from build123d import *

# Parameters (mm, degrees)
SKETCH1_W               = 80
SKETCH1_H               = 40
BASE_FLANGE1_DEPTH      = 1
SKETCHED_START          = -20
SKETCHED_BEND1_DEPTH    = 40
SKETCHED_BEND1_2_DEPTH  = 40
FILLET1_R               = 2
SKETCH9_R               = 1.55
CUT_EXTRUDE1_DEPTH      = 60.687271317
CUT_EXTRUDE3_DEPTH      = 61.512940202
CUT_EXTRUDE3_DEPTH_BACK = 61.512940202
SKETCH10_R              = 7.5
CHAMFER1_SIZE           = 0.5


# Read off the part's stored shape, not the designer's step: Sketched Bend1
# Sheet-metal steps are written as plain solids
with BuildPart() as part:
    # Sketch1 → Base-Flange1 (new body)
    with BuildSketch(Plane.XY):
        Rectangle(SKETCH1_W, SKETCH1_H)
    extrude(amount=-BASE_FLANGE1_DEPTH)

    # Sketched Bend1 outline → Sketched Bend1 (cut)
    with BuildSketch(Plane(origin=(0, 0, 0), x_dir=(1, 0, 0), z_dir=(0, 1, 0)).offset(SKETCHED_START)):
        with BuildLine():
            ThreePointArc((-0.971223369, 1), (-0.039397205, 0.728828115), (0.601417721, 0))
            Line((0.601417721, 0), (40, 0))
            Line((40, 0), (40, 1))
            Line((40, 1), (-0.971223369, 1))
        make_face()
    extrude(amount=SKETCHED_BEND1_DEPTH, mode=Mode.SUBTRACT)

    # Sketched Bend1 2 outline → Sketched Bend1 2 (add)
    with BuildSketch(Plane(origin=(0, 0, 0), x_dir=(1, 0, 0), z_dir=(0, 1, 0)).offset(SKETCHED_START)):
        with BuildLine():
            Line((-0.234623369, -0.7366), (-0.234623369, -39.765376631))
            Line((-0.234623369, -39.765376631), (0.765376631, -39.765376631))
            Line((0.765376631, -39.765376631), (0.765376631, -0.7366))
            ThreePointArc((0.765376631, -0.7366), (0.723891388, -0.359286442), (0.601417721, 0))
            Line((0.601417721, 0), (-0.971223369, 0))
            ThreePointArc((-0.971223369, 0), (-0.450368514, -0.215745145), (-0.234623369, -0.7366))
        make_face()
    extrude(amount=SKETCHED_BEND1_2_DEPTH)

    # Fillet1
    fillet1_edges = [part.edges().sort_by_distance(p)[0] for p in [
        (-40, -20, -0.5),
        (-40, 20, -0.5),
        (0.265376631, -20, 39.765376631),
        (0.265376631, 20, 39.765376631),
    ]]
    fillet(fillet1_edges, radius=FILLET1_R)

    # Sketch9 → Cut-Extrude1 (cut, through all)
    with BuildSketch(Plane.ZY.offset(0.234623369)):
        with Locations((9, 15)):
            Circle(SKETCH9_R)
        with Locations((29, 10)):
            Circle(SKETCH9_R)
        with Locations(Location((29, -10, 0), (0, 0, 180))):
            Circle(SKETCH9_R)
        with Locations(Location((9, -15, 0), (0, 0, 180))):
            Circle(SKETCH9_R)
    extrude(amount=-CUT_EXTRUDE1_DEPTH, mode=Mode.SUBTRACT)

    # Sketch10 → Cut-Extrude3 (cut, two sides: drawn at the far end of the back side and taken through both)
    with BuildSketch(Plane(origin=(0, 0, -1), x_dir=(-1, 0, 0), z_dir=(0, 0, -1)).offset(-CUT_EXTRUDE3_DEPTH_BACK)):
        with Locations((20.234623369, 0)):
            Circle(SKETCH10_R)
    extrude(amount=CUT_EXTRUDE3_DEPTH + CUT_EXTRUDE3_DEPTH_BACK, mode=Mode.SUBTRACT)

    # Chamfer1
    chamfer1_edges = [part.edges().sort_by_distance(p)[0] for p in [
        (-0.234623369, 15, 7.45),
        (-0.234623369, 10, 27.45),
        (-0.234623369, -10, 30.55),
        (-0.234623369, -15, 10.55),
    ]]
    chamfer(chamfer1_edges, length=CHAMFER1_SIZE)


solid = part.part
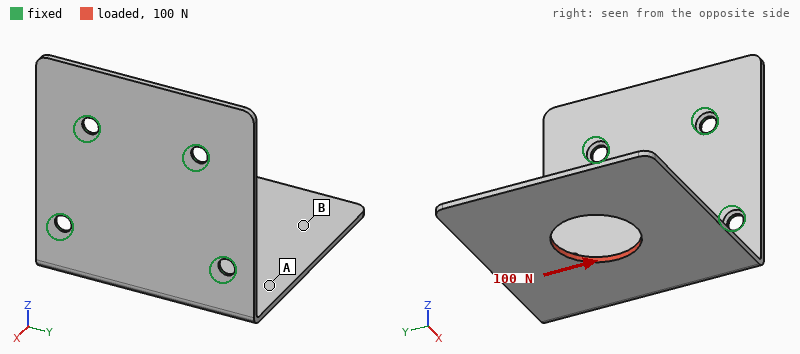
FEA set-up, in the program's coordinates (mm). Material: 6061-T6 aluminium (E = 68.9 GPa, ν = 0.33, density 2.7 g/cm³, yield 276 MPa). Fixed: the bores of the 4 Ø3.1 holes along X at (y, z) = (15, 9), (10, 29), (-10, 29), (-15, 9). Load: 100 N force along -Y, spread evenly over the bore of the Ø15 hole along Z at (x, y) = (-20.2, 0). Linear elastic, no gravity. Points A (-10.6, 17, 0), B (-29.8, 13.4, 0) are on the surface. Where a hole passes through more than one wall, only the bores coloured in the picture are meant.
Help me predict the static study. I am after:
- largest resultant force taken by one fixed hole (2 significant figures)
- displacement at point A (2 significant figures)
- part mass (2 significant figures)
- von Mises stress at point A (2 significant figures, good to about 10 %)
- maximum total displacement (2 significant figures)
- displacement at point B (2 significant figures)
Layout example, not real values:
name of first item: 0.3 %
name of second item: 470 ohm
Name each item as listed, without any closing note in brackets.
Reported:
largest resultant force taken by one fixed hole: 96 N
displacement at point A: 0.23 mm
part mass: 8.1 g
von Mises stress at point A: 33 MPa
maximum total displacement: 0.50 mm
displacement at point B: 0.36 mm
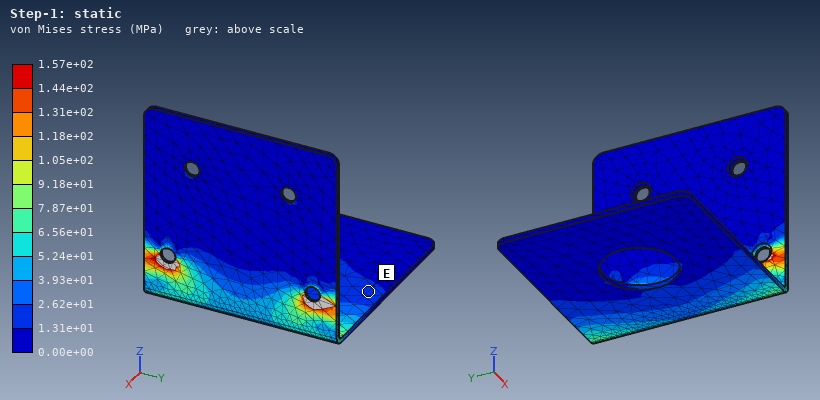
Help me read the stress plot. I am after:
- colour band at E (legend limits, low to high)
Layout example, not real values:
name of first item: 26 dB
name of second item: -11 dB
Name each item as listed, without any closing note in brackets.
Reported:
colour band at E: 1.31e+01 to 2.62e+01 MPa
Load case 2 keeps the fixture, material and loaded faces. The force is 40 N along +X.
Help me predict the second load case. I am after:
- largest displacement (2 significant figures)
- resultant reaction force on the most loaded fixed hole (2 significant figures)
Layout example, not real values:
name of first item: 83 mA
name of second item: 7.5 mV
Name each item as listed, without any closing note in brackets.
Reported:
largest displacement: 0.36 mm
resultant reaction force on the most loaded fixed hole: 28 N
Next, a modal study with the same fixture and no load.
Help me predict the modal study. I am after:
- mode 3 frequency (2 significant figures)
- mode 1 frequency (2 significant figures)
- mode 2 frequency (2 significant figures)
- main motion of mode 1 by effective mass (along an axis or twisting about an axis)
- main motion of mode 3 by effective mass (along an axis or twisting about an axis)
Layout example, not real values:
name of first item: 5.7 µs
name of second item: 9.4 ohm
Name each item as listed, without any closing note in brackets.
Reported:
mode 3 frequency: 1600 Hz
mode 1 frequency: 370 Hz
mode 2 frequency: 990 Hz
main motion of mode 1 by effective mass: along Z
main motion of mode 3 by effective mass: along Y
